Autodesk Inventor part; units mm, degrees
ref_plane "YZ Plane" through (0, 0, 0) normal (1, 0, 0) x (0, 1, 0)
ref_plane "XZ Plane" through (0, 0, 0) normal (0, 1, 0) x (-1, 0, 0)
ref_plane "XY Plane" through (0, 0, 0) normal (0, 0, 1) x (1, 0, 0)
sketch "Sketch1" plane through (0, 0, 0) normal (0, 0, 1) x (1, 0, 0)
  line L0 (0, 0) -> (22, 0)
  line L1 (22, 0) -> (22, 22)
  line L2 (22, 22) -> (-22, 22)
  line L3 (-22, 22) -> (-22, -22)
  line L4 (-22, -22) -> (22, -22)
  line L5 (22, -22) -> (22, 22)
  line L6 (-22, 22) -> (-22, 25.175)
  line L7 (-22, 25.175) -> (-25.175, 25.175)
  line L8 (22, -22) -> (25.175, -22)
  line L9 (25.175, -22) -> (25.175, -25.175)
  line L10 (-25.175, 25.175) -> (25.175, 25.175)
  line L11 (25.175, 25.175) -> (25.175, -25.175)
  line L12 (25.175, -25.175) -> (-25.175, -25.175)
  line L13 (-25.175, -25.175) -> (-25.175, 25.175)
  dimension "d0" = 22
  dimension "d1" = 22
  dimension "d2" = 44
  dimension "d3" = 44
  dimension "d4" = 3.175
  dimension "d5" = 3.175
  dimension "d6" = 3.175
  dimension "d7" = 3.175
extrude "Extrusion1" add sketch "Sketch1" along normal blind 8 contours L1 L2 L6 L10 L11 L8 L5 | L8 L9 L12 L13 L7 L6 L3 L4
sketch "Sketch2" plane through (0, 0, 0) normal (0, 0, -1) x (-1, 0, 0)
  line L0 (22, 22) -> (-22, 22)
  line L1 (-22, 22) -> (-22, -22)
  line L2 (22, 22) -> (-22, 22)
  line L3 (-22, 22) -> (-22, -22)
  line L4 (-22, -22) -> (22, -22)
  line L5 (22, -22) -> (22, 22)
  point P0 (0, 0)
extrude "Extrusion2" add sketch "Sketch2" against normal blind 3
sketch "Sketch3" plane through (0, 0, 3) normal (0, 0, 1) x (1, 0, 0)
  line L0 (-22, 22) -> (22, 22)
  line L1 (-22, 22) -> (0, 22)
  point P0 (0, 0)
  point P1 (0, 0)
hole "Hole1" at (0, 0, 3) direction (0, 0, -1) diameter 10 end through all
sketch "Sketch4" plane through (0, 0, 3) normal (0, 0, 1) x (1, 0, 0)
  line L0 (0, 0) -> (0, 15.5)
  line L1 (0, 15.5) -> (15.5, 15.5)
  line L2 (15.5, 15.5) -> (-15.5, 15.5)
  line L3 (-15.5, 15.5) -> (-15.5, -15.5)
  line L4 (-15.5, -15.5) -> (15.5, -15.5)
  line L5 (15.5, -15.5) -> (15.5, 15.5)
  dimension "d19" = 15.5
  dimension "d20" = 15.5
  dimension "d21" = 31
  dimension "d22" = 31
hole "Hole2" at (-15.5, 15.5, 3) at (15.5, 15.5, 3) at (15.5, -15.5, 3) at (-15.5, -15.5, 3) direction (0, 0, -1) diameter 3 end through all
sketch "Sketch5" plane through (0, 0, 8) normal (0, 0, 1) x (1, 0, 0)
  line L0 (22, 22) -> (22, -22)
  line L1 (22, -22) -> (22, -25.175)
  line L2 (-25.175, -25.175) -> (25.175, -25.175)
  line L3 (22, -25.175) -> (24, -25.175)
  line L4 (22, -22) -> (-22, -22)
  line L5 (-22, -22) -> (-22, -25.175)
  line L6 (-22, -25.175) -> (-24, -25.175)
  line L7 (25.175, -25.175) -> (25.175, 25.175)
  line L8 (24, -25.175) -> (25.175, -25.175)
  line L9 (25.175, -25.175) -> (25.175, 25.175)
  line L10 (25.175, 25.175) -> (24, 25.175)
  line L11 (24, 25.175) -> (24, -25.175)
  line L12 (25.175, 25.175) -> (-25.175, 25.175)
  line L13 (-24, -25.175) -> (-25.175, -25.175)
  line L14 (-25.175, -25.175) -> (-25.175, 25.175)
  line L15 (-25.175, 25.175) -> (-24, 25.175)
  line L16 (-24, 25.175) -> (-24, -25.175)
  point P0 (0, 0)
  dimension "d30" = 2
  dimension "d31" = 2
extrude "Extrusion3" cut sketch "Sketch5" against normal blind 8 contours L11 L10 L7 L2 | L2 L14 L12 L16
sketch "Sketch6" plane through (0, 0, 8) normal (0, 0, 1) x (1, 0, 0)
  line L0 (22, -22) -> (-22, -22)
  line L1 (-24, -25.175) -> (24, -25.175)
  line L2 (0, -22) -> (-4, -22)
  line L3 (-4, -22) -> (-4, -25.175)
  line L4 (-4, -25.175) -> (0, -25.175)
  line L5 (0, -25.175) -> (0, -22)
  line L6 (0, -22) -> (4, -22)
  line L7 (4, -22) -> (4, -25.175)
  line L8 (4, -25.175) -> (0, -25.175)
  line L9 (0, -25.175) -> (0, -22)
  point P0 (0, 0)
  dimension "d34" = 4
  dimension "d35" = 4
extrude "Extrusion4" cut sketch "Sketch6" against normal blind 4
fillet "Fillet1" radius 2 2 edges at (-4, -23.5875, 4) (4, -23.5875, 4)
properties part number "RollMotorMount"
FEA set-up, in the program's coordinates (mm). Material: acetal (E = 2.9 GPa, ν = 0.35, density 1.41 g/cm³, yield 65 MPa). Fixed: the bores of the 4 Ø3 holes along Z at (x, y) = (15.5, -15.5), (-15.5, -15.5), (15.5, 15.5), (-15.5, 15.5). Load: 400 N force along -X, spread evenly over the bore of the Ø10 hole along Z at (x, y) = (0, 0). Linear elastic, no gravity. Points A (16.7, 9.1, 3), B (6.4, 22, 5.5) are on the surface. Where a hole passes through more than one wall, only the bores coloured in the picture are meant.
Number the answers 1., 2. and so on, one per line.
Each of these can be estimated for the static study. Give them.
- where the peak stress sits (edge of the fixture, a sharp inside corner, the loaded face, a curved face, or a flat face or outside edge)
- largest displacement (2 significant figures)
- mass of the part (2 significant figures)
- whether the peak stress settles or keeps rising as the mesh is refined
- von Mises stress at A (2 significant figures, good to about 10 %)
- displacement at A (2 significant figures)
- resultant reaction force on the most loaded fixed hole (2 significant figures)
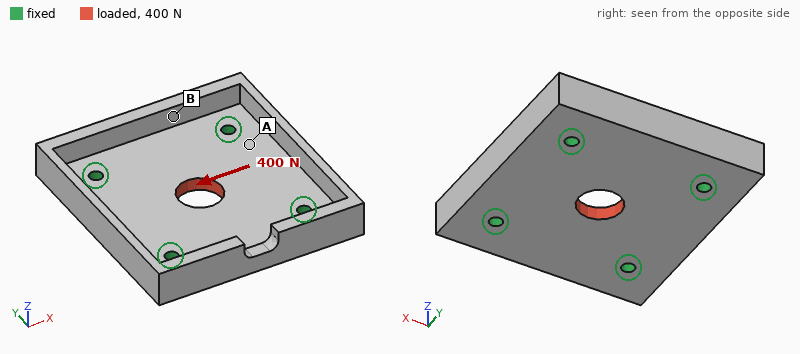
1. edge of the fixture
2. 28 µm
3. 13 g
4. keeps rising
5. 2.3 MPa
6. 11 µm
7. 110 N
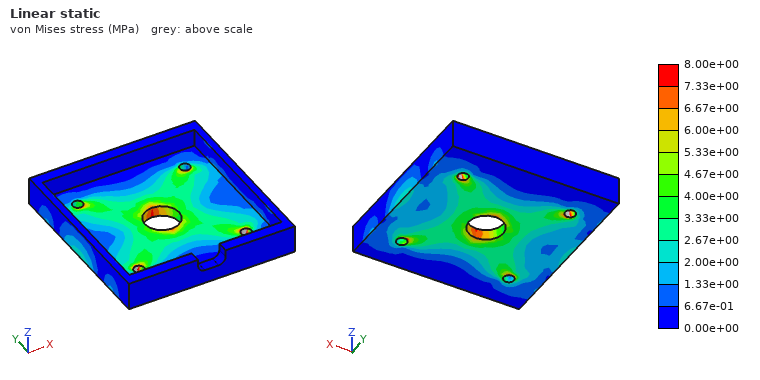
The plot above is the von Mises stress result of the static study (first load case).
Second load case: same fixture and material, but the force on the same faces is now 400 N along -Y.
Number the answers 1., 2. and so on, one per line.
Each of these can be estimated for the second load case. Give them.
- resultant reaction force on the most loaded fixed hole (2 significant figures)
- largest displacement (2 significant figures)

1. 110 N
2. 27 µm
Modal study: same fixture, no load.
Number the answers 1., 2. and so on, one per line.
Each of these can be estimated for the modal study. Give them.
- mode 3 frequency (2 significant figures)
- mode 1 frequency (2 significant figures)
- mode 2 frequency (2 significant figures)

1. 3800 Hz
2. 3400 Hz
3. 3400 Hz
